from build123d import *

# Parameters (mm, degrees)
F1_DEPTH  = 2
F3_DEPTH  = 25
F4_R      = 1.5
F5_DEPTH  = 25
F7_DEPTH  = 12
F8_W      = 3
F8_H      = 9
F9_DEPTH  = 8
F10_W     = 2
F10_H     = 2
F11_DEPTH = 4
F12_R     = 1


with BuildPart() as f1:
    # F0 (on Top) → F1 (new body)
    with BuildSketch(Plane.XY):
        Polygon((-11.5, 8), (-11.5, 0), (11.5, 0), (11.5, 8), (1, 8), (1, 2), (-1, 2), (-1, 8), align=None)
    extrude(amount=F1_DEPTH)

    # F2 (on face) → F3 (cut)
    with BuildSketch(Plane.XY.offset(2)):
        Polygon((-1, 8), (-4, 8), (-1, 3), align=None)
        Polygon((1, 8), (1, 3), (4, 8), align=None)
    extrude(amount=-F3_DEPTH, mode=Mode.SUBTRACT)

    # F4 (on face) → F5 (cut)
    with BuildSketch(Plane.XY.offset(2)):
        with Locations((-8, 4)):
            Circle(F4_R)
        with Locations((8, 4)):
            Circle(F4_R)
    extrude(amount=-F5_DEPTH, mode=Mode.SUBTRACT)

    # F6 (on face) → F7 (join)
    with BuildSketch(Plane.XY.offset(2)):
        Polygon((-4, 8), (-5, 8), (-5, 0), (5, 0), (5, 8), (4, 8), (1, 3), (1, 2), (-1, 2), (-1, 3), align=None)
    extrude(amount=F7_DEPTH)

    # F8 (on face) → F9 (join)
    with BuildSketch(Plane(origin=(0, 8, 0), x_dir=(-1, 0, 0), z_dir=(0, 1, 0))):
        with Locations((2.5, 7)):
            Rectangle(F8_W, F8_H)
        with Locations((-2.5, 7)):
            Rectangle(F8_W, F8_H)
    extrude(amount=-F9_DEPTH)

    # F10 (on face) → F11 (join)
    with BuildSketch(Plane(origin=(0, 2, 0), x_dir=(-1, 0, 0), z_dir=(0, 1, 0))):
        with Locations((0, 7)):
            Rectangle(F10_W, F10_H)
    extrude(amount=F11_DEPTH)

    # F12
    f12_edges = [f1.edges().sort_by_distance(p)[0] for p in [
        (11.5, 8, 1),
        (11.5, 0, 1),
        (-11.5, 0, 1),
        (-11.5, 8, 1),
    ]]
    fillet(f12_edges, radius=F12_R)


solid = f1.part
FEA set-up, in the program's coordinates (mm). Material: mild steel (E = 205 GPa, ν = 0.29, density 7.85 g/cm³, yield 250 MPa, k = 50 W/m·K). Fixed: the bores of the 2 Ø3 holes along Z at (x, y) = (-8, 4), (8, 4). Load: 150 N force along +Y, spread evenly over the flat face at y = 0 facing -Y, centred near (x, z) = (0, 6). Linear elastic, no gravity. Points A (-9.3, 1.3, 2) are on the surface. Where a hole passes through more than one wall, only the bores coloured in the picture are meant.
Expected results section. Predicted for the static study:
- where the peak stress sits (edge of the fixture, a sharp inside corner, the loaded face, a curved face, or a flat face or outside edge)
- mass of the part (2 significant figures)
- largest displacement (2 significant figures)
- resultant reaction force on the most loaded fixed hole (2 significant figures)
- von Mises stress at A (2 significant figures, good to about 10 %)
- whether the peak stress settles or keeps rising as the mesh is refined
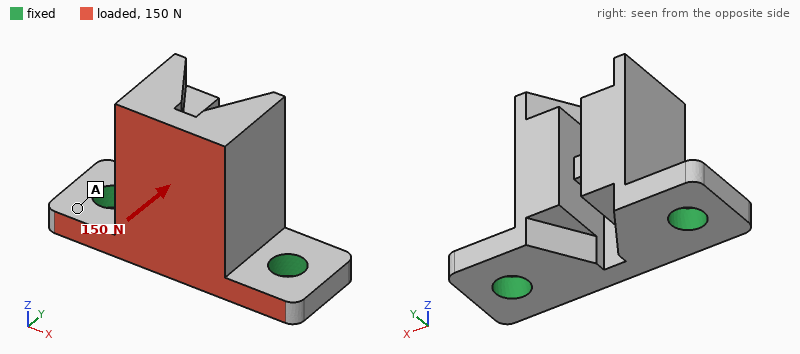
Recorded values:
edge of the fixture
8.4 g
7.6 µm
80 N
11 MPa
keeps rising
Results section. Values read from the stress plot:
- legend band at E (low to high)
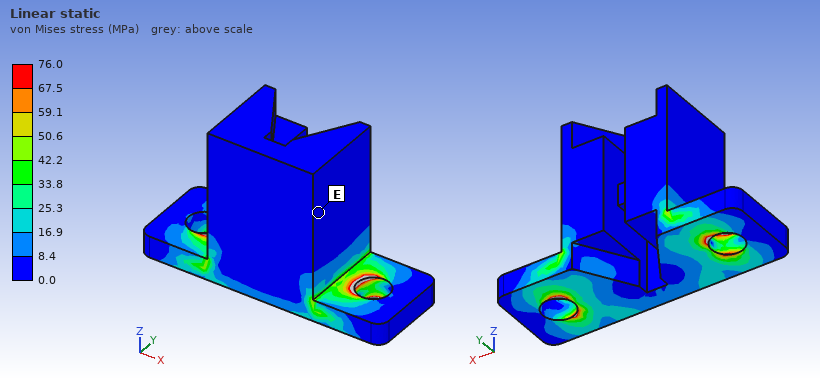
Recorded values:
0.0 to 8.4 MPa
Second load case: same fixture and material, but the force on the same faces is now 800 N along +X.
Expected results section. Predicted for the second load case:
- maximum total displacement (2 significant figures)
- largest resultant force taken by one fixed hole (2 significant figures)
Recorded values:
8.5 µm
570 N
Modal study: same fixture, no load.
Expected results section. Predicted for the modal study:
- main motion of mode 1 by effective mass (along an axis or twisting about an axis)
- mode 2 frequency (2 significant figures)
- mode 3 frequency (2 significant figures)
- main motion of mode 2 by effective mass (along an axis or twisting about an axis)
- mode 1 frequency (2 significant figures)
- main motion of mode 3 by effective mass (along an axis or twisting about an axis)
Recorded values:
along Y
22 kHz
33 kHz
along X
9500 Hz
along Z
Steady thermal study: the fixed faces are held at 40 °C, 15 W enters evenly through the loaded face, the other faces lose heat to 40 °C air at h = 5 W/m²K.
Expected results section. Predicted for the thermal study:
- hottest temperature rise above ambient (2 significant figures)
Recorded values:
58 K
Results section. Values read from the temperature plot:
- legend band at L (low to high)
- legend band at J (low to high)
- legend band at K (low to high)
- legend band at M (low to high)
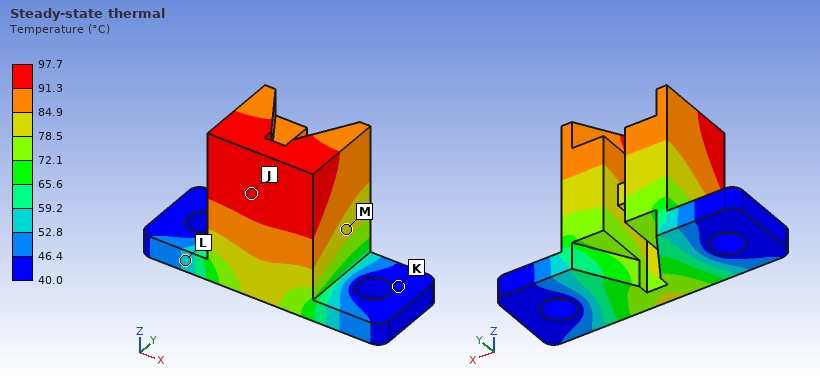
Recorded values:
52.8 to 59.2 °C
91.3 to 97.7 °C
40.0 to 46.4 °C
78.5 to 84.9 °C
